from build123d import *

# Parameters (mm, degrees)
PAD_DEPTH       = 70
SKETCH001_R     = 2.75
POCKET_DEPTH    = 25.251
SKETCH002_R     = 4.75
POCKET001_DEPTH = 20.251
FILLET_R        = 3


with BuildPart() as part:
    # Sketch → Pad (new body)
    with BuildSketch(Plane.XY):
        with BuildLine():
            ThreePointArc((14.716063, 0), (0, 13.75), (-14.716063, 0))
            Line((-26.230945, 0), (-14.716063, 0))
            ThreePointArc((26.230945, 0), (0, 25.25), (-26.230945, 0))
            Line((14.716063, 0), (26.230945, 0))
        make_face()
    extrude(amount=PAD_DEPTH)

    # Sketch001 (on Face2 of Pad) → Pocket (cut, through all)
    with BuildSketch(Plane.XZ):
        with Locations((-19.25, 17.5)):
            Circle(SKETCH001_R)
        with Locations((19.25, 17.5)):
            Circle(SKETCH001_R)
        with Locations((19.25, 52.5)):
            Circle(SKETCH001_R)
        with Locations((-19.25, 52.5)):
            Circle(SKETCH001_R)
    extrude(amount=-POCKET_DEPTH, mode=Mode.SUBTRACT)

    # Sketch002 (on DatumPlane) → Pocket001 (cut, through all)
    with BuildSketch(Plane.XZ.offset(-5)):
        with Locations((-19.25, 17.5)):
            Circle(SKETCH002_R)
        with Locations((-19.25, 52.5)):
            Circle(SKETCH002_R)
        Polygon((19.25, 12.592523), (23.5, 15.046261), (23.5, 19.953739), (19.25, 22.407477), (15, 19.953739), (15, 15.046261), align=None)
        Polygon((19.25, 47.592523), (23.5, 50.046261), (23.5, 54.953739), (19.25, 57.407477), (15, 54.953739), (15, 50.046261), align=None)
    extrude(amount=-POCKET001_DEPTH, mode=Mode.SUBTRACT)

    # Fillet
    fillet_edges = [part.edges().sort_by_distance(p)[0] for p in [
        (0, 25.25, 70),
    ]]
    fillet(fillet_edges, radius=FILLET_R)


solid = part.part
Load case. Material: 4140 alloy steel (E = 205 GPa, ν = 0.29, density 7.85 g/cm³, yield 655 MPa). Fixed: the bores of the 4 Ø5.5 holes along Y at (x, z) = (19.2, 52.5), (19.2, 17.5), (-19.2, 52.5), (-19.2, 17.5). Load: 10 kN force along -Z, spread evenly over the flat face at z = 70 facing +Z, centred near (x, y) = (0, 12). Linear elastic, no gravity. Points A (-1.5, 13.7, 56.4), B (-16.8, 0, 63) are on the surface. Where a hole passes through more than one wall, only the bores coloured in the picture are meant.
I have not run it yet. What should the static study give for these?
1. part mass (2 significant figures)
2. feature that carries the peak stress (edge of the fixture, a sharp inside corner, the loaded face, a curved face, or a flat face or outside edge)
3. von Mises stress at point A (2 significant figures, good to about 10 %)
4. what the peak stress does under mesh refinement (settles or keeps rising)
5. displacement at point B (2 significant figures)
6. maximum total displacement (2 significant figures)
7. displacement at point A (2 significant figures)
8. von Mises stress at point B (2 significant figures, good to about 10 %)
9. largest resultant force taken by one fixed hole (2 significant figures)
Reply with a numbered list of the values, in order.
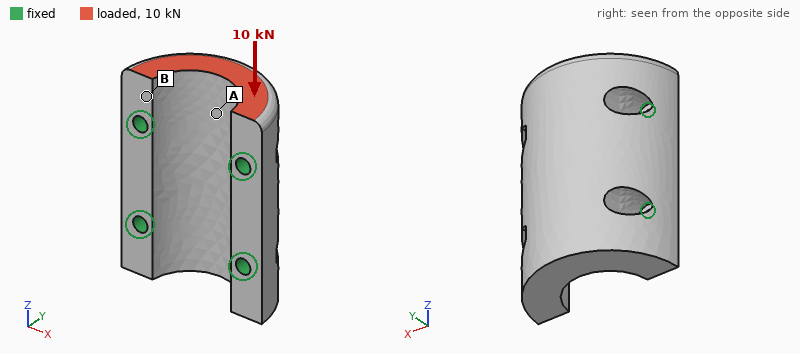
1. 370 g
2. edge of the fixture
3. 15 MPa
4. keeps rising
5. 2.5 µm
6. 6.6 µm
7. 4.4 µm
8. 30 MPa
9. 3.6 kN
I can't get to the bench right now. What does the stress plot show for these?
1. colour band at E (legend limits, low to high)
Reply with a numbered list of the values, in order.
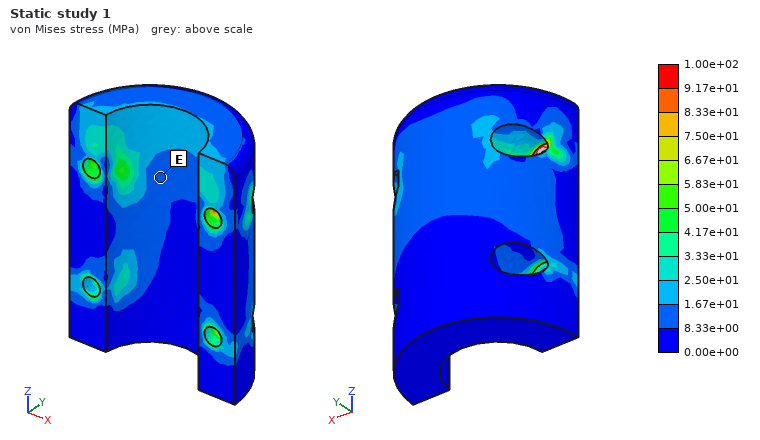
1. 8.33e+00 to 1.67e+01 MPa
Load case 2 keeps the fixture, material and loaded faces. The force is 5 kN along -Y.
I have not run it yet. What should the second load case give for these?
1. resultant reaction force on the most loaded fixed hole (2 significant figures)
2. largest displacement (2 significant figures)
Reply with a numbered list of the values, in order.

1. 3.9 kN
2. 12 µm
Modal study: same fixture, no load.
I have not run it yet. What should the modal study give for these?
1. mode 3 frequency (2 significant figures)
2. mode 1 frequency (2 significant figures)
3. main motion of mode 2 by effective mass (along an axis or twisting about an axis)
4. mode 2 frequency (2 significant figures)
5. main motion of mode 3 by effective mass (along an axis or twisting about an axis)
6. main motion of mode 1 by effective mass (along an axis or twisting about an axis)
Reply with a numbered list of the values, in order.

1. 16 kHz
2. 12 kHz
3. along X
4. 13 kHz
5. twisting about Y
6. along Z
